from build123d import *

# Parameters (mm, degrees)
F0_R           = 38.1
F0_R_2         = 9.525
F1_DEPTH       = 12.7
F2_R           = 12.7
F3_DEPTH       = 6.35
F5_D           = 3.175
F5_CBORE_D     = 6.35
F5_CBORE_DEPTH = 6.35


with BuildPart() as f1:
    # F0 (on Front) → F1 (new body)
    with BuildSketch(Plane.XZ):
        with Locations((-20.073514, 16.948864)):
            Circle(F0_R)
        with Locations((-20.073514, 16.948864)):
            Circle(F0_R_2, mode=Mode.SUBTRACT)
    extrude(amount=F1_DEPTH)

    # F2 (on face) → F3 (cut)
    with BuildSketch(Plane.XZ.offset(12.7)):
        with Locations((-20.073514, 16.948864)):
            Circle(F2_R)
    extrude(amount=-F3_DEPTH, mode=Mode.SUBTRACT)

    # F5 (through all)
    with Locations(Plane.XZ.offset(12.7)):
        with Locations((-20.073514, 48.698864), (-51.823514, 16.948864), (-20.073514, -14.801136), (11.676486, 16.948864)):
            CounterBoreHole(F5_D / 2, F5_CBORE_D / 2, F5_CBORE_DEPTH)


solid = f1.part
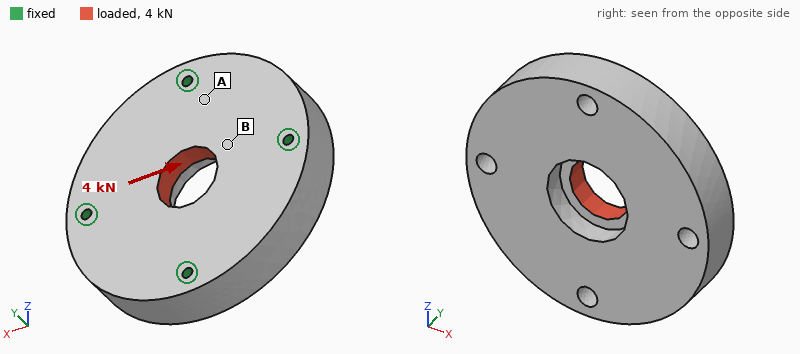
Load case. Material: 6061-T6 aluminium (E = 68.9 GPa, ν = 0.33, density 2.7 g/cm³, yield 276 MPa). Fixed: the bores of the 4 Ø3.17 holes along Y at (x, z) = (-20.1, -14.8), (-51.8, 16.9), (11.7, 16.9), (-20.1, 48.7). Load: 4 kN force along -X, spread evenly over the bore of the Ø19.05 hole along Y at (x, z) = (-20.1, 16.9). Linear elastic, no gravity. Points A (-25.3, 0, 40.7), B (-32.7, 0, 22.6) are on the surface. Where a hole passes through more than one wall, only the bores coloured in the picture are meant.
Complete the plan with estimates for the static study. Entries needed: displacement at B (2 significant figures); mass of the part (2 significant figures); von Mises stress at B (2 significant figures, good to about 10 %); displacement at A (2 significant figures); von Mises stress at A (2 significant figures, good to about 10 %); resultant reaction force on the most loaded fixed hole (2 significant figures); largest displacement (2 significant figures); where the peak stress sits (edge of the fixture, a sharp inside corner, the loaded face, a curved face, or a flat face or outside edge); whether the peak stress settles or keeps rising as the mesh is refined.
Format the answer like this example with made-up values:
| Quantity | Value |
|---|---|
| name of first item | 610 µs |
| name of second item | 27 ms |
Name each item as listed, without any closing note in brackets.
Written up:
| Quantity | Value |
|---|---|
| displacement at B | 3.2 µm |
| mass of the part | 140 g |
| von Mises stress at B | 11 MPa |
| displacement at A | 1.5 µm |
| von Mises stress at A | 3.2 MPa |
| resultant reaction force on the most loaded fixed hole | 1.2 kN |
| largest displacement | 4.0 µm |
| where the peak stress sits | edge of the fixture |
| whether the peak stress settles or keeps rising as the mesh is refined | keeps rising |
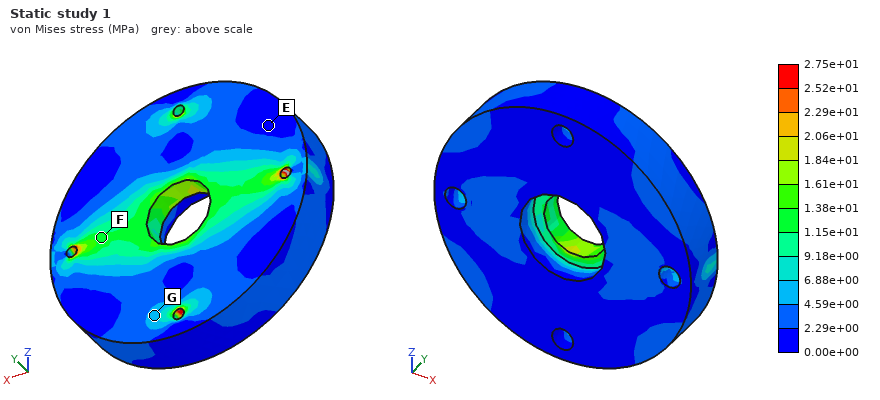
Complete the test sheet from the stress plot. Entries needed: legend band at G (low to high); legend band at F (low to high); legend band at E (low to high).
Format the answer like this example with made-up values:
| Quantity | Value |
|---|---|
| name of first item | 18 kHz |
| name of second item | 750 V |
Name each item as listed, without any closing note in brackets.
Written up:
| Quantity | Value |
|---|---|
| legend band at G | 4.59e+00 to 6.88e+00 MPa |
| legend band at F | 1.15e+01 to 1.38e+01 MPa |
| legend band at E | 0.00e+00 to 2.29e+00 MPa |
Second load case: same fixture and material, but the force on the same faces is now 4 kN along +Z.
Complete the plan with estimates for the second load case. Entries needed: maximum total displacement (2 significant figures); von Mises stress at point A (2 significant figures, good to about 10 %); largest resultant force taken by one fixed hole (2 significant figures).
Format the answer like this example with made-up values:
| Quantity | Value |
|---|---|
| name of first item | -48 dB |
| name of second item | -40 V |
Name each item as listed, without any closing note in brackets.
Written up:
| Quantity | Value |
|---|---|
| maximum total displacement | 4.0 µm |
| von Mises stress at point A | 9.0 MPa |
| largest resultant force taken by one fixed hole | 1.2 kN |
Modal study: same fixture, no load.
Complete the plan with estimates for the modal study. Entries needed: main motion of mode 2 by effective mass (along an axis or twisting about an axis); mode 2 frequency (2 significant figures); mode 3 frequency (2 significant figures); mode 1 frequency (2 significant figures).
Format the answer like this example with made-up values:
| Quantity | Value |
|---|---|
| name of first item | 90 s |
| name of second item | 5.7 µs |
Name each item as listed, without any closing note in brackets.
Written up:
| Quantity | Value |
|---|---|
| main motion of mode 2 by effective mass | along Y |
| mode 2 frequency | 13 kHz |
| mode 3 frequency | 14 kHz |
| mode 1 frequency | 12 kHz |
